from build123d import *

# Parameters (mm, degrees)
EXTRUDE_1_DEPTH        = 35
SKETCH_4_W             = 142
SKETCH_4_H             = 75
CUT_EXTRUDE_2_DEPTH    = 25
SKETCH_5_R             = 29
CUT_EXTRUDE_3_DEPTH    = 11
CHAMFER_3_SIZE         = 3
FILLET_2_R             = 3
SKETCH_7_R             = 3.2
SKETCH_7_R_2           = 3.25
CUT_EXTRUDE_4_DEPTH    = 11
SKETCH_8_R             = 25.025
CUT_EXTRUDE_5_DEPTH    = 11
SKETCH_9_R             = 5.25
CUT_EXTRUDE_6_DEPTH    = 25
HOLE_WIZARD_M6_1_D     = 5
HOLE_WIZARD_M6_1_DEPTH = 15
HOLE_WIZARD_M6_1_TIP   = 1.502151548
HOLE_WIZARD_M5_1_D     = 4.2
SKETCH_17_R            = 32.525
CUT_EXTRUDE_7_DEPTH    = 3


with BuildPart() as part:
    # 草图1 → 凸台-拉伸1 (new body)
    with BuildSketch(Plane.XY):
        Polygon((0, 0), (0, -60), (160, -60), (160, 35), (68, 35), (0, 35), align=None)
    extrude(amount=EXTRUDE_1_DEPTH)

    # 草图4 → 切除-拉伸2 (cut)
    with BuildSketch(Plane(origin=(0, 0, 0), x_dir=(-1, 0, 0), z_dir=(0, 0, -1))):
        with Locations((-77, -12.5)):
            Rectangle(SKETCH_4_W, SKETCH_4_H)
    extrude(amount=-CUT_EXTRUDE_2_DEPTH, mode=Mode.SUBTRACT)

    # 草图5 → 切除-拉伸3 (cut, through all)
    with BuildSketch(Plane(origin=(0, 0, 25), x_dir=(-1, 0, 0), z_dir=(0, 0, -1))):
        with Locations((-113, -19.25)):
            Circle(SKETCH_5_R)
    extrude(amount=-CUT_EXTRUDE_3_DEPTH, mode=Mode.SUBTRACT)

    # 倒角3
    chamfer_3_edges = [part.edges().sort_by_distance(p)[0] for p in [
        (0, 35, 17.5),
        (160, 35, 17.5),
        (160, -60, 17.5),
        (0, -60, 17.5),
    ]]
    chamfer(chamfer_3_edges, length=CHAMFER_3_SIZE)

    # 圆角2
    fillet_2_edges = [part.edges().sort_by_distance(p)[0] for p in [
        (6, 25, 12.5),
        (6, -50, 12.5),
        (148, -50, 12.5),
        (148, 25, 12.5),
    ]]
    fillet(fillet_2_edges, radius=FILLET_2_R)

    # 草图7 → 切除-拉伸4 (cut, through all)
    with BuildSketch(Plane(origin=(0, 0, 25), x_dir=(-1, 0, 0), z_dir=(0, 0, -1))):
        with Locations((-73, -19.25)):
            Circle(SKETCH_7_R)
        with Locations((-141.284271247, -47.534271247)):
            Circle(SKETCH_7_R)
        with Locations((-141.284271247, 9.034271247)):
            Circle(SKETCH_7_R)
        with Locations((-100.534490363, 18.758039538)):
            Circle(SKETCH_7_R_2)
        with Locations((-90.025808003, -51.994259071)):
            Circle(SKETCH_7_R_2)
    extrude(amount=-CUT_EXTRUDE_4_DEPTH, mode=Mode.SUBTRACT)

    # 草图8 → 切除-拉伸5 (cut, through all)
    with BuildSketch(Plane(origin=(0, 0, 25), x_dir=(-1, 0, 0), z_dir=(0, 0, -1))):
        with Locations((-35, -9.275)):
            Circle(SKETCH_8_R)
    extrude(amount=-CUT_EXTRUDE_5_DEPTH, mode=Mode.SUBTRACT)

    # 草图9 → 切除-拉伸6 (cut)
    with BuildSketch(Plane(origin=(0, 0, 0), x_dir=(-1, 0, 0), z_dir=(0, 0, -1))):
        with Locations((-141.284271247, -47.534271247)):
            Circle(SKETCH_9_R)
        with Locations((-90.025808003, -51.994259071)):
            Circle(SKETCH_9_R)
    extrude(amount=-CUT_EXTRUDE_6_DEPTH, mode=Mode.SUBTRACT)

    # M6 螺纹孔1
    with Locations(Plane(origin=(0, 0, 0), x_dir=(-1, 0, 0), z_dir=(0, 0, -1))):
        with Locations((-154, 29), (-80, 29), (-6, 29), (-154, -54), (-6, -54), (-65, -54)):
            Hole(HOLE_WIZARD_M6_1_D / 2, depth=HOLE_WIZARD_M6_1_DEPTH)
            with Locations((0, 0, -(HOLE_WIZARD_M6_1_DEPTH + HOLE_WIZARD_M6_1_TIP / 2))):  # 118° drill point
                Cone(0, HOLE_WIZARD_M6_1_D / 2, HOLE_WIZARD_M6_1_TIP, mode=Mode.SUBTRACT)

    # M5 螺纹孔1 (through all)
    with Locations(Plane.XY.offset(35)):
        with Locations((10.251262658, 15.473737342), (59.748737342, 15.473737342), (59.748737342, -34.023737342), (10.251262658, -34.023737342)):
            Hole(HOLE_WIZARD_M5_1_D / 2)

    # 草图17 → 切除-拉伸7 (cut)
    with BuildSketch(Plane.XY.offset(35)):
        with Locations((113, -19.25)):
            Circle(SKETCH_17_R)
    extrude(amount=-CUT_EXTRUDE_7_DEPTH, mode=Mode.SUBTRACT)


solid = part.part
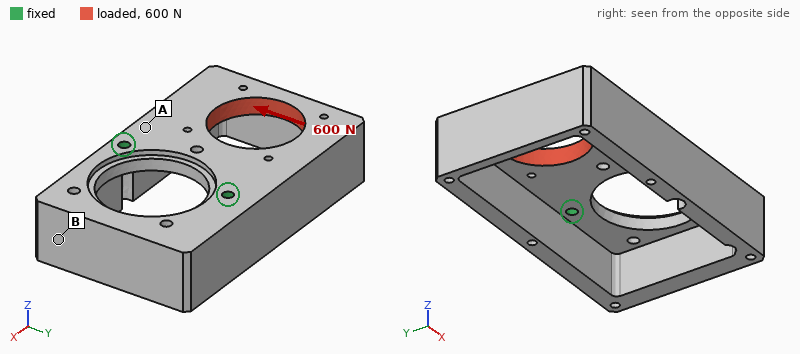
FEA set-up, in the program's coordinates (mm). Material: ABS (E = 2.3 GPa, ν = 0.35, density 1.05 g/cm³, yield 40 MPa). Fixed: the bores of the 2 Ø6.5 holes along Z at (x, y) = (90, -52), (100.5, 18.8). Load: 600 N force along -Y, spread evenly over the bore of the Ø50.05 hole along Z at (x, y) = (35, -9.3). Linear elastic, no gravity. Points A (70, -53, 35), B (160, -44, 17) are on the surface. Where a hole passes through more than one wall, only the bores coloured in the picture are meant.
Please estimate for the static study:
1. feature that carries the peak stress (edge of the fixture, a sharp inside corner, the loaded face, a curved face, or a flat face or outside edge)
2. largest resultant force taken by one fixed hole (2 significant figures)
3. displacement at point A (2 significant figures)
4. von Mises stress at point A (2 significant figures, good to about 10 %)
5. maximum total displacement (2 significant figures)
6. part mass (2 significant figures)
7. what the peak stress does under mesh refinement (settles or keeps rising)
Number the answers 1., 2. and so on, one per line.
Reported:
1. edge of the fixture
2. 570 N
3. 0.050 mm
4. 1.6 MPa
5. 0.30 mm
6. 220 g
7. keeps rising
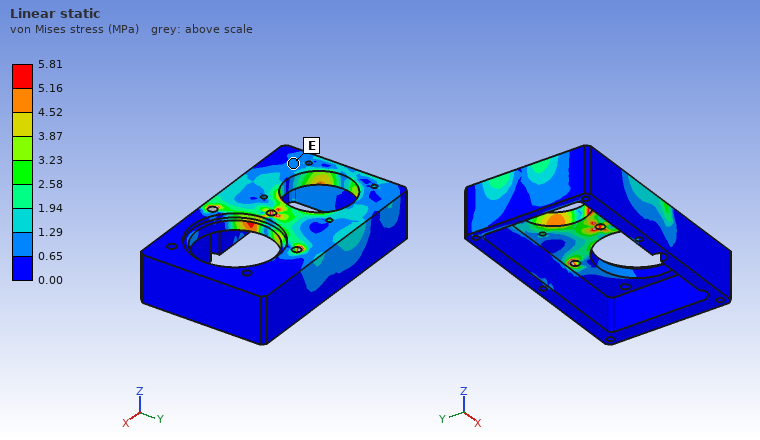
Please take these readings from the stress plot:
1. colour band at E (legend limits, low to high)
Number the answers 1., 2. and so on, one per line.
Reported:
1. 0.65 to 1.29 MPa
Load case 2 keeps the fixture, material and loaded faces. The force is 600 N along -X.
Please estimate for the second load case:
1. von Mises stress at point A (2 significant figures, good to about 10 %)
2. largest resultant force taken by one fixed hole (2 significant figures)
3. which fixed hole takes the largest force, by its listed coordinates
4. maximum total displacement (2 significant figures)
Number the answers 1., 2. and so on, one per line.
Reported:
1. 1.1 MPa
2. 370 N
3. (100.5, 18.8)
4. 91 µm
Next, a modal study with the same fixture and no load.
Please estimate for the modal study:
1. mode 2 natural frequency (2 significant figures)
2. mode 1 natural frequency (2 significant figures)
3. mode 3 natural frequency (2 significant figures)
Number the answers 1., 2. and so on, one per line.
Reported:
1. 470 Hz
2. 260 Hz
3. 700 Hz
